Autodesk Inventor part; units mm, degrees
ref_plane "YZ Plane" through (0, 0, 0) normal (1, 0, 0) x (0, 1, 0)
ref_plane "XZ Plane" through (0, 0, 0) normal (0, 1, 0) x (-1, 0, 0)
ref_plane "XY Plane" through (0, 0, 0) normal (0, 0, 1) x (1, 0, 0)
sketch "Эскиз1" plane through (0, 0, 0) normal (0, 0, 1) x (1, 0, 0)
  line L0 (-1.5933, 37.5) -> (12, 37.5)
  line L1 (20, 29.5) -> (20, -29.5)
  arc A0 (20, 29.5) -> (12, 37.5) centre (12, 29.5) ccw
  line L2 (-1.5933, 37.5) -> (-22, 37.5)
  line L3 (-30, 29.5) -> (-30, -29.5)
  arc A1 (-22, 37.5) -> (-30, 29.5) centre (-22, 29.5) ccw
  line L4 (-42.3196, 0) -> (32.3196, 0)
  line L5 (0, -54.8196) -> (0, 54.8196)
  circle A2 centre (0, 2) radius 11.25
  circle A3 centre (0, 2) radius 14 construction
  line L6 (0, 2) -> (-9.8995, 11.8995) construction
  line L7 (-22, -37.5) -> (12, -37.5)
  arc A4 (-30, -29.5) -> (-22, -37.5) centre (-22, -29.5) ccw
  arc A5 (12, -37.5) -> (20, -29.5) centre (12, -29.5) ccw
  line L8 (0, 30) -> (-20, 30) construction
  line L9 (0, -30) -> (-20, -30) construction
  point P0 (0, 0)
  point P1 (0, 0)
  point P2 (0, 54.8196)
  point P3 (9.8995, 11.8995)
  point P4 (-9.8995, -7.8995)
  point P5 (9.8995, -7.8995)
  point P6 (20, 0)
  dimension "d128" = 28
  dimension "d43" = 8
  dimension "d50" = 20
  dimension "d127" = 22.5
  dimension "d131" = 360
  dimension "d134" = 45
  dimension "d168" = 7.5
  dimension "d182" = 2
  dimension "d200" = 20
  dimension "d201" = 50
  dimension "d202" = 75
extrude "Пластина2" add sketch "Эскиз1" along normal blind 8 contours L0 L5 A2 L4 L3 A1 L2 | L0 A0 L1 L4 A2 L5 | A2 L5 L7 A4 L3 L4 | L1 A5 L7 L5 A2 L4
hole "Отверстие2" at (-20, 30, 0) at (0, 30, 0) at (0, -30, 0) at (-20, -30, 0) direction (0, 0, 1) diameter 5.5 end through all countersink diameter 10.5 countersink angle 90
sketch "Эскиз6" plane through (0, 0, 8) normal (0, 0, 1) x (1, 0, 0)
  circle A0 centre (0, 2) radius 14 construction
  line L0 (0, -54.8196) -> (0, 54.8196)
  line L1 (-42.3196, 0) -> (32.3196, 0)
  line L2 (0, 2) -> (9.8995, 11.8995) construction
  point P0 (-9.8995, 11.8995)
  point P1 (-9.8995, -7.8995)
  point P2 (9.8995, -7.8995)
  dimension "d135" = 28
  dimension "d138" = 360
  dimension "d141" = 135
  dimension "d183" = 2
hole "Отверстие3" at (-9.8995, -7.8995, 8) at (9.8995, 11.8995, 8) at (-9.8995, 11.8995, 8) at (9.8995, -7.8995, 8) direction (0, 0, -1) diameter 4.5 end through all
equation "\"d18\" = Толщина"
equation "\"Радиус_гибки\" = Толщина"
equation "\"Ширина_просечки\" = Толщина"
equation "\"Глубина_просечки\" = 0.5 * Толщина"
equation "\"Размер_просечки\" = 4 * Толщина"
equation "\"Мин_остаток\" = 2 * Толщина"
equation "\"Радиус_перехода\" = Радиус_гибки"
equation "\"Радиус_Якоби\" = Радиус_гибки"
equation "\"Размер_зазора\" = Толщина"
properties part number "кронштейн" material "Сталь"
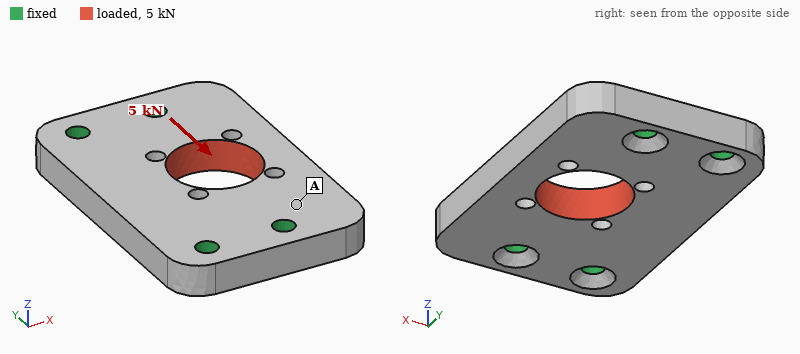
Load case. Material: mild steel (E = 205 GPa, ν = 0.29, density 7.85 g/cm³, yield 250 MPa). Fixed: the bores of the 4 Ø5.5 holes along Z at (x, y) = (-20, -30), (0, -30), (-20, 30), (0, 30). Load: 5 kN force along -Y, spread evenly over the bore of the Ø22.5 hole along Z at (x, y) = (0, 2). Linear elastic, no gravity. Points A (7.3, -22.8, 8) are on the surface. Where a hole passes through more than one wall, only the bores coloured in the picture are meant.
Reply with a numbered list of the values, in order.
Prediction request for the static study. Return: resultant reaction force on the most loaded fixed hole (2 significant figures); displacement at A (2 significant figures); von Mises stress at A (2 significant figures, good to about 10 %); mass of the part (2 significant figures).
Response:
1. 1.9 kN
2. 1.1 µm
3. 12 MPa
4. 190 g
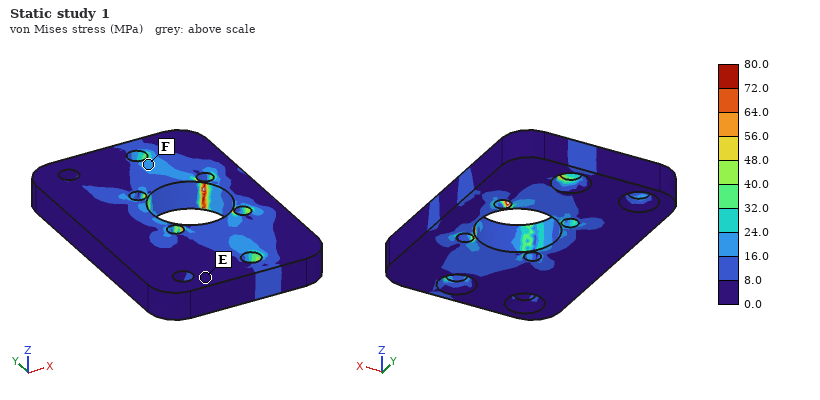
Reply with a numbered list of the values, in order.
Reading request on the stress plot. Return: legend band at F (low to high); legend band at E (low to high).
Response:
1. 16.0 to 24.0 MPa
2. 0.0 to 8.0 MPa
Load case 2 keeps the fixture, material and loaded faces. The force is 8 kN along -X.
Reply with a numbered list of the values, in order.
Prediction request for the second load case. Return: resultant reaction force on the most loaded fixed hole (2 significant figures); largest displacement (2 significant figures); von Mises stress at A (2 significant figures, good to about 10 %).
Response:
1. 2.5 kN
2. 8.3 µm
3. 16 MPa
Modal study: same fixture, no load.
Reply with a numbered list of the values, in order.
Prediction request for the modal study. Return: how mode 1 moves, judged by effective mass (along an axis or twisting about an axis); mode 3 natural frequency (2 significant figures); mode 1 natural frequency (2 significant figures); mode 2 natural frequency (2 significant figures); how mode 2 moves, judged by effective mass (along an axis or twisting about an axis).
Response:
1. along Z
2. 14 kHz
3. 7900 Hz
4. 10 kHz
5. along Z
